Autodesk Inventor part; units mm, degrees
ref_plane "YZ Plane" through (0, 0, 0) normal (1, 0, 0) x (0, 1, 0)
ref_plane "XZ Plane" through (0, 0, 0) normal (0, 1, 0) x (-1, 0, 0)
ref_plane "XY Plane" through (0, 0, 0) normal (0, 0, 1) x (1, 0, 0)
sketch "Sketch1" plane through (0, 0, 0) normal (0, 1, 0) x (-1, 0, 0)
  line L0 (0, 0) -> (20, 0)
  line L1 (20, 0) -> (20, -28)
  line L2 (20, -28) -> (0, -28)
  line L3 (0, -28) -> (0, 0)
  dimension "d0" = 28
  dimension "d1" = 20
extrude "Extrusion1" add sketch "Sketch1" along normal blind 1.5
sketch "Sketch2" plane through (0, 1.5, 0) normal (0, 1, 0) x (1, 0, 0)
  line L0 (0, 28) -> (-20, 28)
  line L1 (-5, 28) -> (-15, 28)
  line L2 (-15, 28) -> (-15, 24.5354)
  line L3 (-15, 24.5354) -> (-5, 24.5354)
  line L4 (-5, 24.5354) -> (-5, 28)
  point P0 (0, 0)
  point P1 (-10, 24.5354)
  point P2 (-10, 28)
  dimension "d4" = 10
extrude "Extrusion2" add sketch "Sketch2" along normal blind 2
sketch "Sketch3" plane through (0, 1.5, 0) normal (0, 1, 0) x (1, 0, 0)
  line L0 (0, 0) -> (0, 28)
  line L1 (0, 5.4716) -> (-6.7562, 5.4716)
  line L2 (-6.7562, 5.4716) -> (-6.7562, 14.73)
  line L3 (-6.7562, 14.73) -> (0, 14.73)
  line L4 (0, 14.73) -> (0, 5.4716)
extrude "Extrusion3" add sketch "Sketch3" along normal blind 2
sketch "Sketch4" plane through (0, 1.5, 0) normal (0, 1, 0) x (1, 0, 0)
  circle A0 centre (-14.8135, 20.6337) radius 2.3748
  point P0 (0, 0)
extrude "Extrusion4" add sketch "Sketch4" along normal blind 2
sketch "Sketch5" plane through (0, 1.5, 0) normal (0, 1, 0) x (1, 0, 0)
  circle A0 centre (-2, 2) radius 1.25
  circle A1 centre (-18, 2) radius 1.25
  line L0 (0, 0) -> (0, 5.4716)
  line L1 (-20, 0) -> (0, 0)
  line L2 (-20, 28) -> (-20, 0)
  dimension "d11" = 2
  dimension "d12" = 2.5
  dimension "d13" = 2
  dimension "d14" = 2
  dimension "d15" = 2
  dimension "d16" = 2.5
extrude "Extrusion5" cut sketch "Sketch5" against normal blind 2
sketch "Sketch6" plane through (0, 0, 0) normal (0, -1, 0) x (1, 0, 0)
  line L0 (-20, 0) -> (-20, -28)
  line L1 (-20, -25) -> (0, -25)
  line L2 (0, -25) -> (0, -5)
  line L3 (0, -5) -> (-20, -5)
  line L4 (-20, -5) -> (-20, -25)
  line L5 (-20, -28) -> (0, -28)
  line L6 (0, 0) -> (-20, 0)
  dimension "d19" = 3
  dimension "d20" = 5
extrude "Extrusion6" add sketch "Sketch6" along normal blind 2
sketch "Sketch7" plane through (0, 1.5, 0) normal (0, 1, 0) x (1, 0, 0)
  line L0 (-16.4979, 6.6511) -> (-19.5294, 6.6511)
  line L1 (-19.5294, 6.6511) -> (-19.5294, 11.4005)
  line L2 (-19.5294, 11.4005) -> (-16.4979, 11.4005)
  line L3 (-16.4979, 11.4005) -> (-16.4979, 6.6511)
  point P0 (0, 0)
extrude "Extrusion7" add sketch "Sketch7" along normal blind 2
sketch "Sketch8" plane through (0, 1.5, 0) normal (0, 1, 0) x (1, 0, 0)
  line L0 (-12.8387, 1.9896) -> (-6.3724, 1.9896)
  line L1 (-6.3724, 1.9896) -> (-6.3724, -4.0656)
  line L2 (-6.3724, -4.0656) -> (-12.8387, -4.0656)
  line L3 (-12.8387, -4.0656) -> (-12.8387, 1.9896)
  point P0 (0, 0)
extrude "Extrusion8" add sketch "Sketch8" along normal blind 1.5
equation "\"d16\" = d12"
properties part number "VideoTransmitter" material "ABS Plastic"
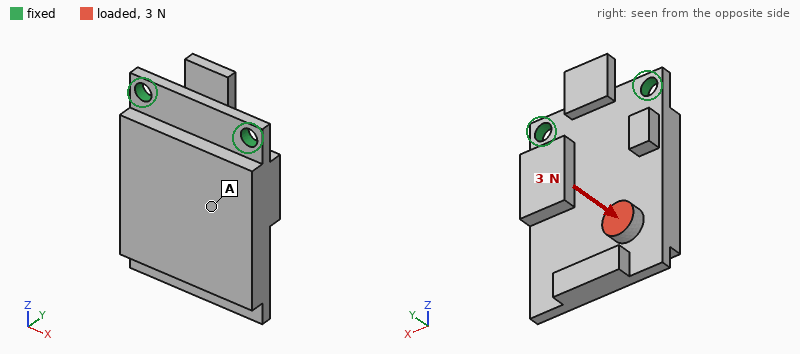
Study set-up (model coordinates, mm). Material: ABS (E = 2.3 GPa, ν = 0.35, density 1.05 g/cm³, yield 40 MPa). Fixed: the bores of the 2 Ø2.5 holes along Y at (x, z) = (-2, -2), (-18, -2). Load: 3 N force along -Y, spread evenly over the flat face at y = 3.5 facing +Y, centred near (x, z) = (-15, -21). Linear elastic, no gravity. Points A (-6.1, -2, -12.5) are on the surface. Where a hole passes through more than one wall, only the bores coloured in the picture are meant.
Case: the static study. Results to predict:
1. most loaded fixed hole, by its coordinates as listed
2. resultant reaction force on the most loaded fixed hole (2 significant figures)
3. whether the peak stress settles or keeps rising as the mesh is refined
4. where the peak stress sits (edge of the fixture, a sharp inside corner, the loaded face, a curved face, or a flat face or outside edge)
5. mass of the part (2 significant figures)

(-18, -2)
2.7 N
keeps rising
edge of the fixture
2.0 g
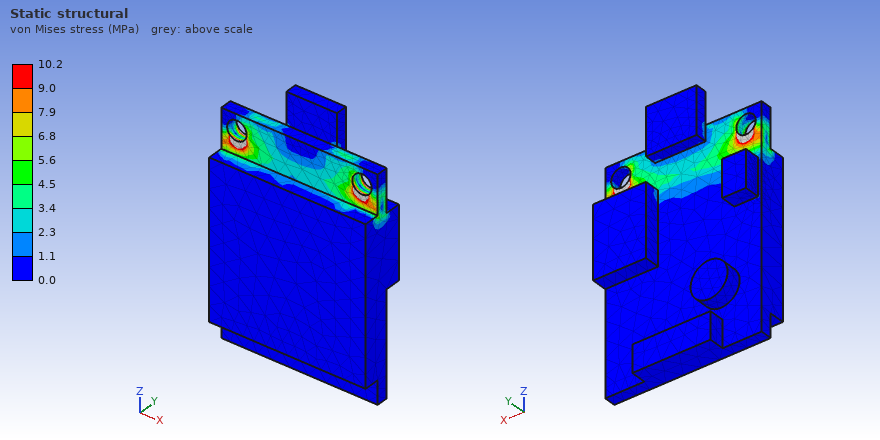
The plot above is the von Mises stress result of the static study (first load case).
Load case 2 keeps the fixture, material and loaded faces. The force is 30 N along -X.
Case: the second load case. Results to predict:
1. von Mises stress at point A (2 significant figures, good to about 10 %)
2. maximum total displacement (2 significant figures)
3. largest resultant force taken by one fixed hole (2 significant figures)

1.4 MPa
0.13 mm
37 N
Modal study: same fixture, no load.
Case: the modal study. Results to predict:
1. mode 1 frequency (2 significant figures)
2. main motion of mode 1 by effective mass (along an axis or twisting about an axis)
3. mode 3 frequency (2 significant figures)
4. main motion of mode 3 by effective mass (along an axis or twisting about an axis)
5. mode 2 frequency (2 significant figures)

510 Hz
along Y
4500 Hz
along X
3000 Hz
